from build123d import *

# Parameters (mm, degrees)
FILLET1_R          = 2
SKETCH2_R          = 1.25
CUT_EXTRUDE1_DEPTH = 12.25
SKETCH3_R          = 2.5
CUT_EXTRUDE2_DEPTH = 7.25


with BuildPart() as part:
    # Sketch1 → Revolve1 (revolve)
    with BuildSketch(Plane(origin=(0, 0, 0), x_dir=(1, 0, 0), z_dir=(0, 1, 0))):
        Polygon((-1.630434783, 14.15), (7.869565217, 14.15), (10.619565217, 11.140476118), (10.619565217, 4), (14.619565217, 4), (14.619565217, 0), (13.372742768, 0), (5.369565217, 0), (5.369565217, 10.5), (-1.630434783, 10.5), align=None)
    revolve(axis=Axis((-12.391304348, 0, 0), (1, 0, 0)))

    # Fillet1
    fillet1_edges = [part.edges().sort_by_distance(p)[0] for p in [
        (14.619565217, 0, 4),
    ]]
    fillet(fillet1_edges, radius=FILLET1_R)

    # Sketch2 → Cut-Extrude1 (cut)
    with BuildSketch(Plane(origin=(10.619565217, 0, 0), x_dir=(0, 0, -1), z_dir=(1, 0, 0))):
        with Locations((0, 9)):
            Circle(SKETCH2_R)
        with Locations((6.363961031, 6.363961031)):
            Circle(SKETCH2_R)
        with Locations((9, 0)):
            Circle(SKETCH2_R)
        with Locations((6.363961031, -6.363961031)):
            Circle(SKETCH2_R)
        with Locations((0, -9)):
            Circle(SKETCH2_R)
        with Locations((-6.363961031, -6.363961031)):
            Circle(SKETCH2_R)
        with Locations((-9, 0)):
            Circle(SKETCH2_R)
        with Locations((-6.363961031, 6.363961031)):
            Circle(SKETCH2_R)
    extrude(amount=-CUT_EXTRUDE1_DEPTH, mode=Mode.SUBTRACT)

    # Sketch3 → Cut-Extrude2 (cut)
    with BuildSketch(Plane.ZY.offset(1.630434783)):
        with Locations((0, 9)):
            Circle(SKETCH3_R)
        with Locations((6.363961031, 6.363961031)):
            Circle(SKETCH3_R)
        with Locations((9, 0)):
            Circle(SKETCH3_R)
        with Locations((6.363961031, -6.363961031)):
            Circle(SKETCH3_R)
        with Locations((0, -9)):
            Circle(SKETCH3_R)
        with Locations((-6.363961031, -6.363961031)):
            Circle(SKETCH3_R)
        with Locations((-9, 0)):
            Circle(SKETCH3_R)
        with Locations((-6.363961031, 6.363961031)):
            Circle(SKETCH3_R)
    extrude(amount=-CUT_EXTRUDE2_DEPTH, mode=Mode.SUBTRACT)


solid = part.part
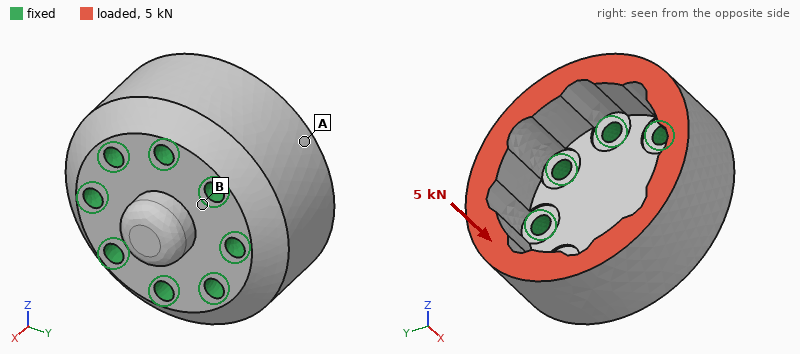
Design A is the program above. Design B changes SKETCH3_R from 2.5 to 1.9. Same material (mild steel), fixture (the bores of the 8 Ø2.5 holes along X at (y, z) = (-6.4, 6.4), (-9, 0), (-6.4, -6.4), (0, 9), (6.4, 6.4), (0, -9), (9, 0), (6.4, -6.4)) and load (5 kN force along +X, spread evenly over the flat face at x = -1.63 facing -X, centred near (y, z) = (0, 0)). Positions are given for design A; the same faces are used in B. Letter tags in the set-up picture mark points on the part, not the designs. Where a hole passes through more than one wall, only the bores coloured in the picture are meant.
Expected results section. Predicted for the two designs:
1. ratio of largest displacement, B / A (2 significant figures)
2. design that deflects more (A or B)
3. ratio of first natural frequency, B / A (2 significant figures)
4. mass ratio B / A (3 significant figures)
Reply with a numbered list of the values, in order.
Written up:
1. 0.91
2. A
3. 1.0
4. 1.03
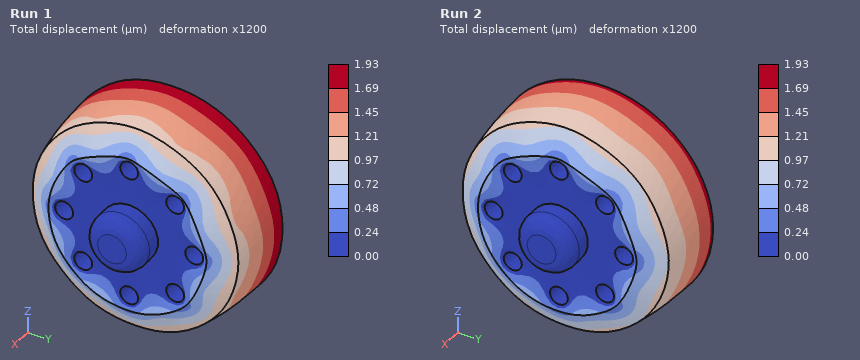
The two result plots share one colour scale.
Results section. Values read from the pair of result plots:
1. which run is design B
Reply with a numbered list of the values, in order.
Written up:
1. Run 2
